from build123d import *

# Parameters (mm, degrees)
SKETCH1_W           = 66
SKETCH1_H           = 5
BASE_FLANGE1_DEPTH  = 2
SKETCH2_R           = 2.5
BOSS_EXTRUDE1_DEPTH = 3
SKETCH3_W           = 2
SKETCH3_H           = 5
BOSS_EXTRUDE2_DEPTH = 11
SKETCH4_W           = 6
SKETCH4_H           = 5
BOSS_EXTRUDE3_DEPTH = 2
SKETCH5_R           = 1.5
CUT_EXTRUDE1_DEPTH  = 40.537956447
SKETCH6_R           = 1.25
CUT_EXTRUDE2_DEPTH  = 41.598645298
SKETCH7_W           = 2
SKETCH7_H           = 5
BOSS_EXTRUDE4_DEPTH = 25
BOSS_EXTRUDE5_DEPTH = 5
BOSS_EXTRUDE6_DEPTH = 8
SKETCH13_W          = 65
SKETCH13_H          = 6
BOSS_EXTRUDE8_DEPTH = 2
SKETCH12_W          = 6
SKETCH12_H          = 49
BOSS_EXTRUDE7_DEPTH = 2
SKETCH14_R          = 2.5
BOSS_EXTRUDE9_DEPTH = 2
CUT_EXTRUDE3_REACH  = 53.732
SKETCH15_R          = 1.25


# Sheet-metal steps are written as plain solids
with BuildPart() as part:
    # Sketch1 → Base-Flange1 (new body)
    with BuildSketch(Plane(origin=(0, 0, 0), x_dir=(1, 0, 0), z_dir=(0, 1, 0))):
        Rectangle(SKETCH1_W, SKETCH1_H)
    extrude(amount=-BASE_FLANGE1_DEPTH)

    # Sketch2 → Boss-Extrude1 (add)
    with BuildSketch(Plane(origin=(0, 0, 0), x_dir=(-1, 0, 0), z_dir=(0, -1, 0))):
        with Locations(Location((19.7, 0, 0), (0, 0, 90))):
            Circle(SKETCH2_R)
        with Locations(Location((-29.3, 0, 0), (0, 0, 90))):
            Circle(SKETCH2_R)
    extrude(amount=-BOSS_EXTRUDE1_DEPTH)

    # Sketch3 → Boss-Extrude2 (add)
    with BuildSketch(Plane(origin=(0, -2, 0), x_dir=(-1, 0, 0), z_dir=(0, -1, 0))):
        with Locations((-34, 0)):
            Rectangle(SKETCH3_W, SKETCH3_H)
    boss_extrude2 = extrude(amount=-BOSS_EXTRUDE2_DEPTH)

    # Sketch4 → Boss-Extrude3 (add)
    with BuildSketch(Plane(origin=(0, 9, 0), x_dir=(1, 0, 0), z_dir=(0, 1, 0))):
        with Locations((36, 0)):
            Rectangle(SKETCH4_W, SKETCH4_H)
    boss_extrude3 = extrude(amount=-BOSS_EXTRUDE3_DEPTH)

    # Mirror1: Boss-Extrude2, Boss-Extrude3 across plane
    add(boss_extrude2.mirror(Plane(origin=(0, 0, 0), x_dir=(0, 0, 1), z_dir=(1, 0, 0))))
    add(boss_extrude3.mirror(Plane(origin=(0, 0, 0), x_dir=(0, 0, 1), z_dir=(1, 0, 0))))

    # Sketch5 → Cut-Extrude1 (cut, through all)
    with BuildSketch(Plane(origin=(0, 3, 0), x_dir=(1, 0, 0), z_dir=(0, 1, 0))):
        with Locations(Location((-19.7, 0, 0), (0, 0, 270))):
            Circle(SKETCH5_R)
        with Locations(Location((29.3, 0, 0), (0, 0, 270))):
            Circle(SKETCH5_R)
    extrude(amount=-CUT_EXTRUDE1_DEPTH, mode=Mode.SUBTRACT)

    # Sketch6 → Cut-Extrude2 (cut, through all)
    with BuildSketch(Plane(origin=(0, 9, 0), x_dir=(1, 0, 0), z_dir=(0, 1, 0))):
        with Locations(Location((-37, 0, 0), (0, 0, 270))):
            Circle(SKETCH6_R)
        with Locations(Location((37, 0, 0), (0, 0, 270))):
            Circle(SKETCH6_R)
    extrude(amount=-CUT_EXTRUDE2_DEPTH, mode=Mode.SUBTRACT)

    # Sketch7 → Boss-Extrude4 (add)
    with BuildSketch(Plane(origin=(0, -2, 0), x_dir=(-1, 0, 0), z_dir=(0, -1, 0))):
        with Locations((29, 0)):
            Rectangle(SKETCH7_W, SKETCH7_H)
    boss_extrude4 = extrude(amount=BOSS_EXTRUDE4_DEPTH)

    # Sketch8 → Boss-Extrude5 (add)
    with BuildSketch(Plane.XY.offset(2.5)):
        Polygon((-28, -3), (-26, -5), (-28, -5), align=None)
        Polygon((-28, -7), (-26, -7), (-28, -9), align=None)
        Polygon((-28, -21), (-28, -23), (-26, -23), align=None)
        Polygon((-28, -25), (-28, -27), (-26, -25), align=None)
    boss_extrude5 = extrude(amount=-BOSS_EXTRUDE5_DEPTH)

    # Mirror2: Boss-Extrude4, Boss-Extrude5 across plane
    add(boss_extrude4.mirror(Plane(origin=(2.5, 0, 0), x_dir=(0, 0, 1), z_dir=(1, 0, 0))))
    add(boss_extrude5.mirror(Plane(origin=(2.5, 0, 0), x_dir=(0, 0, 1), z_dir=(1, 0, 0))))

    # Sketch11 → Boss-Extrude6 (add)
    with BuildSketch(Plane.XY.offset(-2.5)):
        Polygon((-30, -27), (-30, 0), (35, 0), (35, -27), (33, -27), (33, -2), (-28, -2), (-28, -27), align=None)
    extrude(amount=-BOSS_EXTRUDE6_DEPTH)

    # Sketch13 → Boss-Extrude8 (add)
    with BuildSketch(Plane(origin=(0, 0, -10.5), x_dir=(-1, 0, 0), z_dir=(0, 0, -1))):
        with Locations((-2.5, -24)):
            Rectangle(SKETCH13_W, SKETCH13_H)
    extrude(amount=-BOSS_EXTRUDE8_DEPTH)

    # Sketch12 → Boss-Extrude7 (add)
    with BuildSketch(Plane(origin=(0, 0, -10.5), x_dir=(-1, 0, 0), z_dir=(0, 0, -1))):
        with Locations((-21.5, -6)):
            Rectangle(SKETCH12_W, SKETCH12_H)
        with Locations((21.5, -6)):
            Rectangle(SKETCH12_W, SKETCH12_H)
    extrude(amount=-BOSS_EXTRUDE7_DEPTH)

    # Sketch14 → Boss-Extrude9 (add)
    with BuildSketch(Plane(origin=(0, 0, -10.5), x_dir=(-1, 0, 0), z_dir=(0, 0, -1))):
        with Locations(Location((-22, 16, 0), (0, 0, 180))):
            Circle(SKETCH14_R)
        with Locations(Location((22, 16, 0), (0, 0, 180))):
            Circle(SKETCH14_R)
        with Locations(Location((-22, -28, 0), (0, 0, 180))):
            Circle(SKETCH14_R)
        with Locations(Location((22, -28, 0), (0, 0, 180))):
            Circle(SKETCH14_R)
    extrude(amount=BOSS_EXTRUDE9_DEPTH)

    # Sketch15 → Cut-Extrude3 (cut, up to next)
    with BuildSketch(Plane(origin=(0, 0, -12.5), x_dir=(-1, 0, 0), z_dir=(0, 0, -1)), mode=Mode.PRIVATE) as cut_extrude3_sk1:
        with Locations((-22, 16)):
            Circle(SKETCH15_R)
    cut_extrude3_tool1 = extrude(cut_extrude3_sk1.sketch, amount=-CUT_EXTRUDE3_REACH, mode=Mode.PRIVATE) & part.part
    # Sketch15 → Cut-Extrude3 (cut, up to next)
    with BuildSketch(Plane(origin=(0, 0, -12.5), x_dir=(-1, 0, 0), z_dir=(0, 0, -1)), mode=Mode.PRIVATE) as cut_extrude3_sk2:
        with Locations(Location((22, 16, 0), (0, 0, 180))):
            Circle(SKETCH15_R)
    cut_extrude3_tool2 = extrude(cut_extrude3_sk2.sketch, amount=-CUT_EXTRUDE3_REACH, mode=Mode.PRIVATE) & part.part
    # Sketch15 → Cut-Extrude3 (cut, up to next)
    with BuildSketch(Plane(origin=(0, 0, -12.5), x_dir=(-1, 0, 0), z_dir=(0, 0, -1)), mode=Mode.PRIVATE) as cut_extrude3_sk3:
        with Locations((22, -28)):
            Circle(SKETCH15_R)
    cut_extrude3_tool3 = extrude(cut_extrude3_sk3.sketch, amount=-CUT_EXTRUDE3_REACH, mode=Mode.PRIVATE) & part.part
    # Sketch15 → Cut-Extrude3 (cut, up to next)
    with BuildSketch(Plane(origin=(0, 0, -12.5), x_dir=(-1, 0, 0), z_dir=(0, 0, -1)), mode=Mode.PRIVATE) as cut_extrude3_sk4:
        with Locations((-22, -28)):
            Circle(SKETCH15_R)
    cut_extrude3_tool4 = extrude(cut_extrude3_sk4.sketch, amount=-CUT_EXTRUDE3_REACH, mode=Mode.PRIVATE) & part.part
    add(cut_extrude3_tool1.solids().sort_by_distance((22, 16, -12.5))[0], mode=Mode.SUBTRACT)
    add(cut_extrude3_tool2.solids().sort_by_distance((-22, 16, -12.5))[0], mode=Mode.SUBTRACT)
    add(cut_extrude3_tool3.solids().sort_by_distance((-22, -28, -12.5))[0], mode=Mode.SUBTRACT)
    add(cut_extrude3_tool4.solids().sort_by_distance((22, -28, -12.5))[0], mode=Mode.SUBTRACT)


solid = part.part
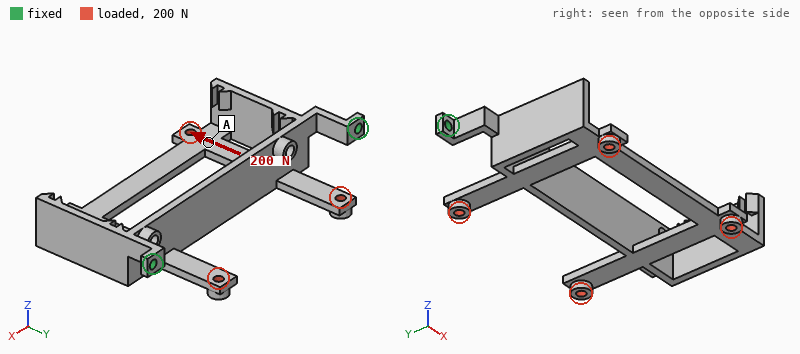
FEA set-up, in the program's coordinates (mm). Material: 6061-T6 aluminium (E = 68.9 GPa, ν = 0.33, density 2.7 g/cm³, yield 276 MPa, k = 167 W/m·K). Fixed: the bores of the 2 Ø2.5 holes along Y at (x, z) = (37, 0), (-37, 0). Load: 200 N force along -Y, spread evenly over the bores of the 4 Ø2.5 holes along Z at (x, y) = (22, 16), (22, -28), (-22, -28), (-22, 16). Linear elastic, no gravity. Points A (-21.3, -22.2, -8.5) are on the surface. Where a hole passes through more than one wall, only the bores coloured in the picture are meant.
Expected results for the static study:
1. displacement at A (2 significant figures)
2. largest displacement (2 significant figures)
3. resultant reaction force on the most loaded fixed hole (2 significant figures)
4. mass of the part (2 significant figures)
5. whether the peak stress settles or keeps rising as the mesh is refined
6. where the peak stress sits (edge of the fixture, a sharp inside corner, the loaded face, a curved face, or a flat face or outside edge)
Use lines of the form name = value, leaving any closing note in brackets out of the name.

displacement at A = 0.53 mm
largest displacement = 0.71 mm
resultant reaction force on the most loaded fixed hole = 110 N
mass of the part = 14 g
whether the peak stress settles or keeps rising as the mesh is refined = keeps rising
where the peak stress sits = edge of the fixture
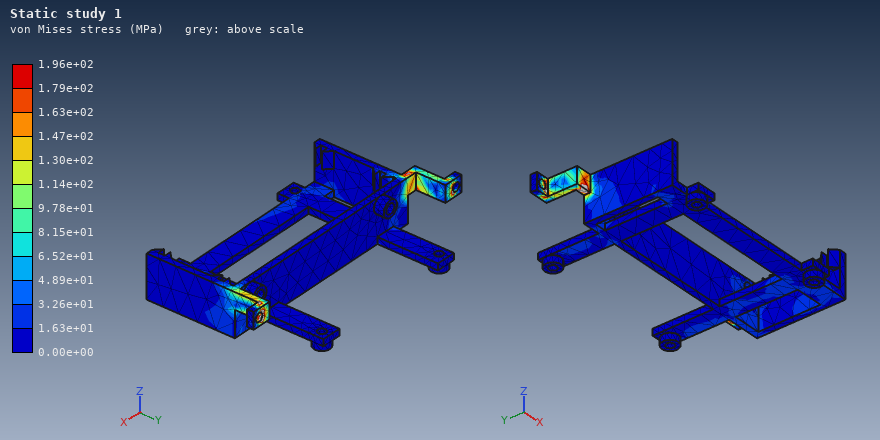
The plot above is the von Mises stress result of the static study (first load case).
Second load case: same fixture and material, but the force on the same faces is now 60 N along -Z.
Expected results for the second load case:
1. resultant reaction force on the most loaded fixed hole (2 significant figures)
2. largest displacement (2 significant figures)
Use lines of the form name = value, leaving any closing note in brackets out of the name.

resultant reaction force on the most loaded fixed hole = 30 N
largest displacement = 0.21 mm
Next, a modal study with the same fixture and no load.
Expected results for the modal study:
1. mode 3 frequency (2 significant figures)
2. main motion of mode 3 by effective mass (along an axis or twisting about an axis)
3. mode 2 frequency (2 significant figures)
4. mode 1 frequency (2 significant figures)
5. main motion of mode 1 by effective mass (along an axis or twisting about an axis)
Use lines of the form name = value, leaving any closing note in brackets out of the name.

mode 3 frequency = 2100 Hz
main motion of mode 3 by effective mass = along X
mode 2 frequency = 1400 Hz
mode 1 frequency = 810 Hz
main motion of mode 1 by effective mass = along Z
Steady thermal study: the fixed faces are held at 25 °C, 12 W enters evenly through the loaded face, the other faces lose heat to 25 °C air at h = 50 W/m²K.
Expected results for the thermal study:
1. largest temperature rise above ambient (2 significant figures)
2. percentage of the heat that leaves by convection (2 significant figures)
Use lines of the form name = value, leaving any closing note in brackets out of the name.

largest temperature rise above ambient = 46 K
percentage of the heat that leaves by convection = 62 %
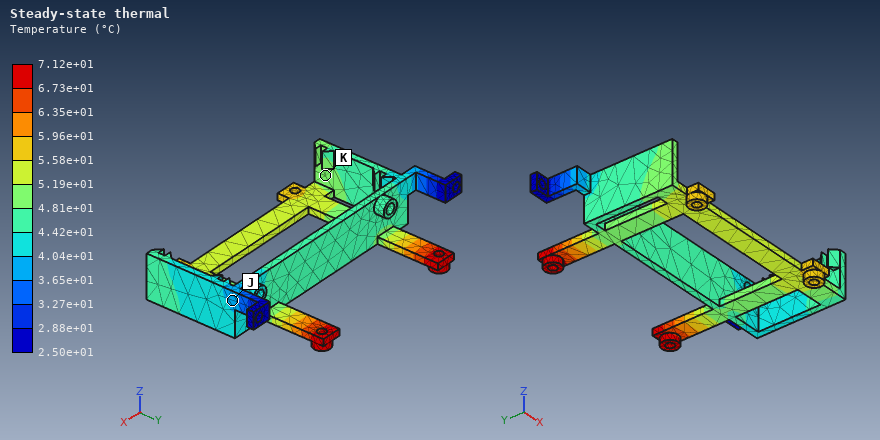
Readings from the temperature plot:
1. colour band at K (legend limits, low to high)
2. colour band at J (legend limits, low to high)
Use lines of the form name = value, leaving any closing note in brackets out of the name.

colour band at K = 4.81e+01 to 5.19e+01 °C
colour band at J = 3.65e+01 to 4.04e+01 °C
